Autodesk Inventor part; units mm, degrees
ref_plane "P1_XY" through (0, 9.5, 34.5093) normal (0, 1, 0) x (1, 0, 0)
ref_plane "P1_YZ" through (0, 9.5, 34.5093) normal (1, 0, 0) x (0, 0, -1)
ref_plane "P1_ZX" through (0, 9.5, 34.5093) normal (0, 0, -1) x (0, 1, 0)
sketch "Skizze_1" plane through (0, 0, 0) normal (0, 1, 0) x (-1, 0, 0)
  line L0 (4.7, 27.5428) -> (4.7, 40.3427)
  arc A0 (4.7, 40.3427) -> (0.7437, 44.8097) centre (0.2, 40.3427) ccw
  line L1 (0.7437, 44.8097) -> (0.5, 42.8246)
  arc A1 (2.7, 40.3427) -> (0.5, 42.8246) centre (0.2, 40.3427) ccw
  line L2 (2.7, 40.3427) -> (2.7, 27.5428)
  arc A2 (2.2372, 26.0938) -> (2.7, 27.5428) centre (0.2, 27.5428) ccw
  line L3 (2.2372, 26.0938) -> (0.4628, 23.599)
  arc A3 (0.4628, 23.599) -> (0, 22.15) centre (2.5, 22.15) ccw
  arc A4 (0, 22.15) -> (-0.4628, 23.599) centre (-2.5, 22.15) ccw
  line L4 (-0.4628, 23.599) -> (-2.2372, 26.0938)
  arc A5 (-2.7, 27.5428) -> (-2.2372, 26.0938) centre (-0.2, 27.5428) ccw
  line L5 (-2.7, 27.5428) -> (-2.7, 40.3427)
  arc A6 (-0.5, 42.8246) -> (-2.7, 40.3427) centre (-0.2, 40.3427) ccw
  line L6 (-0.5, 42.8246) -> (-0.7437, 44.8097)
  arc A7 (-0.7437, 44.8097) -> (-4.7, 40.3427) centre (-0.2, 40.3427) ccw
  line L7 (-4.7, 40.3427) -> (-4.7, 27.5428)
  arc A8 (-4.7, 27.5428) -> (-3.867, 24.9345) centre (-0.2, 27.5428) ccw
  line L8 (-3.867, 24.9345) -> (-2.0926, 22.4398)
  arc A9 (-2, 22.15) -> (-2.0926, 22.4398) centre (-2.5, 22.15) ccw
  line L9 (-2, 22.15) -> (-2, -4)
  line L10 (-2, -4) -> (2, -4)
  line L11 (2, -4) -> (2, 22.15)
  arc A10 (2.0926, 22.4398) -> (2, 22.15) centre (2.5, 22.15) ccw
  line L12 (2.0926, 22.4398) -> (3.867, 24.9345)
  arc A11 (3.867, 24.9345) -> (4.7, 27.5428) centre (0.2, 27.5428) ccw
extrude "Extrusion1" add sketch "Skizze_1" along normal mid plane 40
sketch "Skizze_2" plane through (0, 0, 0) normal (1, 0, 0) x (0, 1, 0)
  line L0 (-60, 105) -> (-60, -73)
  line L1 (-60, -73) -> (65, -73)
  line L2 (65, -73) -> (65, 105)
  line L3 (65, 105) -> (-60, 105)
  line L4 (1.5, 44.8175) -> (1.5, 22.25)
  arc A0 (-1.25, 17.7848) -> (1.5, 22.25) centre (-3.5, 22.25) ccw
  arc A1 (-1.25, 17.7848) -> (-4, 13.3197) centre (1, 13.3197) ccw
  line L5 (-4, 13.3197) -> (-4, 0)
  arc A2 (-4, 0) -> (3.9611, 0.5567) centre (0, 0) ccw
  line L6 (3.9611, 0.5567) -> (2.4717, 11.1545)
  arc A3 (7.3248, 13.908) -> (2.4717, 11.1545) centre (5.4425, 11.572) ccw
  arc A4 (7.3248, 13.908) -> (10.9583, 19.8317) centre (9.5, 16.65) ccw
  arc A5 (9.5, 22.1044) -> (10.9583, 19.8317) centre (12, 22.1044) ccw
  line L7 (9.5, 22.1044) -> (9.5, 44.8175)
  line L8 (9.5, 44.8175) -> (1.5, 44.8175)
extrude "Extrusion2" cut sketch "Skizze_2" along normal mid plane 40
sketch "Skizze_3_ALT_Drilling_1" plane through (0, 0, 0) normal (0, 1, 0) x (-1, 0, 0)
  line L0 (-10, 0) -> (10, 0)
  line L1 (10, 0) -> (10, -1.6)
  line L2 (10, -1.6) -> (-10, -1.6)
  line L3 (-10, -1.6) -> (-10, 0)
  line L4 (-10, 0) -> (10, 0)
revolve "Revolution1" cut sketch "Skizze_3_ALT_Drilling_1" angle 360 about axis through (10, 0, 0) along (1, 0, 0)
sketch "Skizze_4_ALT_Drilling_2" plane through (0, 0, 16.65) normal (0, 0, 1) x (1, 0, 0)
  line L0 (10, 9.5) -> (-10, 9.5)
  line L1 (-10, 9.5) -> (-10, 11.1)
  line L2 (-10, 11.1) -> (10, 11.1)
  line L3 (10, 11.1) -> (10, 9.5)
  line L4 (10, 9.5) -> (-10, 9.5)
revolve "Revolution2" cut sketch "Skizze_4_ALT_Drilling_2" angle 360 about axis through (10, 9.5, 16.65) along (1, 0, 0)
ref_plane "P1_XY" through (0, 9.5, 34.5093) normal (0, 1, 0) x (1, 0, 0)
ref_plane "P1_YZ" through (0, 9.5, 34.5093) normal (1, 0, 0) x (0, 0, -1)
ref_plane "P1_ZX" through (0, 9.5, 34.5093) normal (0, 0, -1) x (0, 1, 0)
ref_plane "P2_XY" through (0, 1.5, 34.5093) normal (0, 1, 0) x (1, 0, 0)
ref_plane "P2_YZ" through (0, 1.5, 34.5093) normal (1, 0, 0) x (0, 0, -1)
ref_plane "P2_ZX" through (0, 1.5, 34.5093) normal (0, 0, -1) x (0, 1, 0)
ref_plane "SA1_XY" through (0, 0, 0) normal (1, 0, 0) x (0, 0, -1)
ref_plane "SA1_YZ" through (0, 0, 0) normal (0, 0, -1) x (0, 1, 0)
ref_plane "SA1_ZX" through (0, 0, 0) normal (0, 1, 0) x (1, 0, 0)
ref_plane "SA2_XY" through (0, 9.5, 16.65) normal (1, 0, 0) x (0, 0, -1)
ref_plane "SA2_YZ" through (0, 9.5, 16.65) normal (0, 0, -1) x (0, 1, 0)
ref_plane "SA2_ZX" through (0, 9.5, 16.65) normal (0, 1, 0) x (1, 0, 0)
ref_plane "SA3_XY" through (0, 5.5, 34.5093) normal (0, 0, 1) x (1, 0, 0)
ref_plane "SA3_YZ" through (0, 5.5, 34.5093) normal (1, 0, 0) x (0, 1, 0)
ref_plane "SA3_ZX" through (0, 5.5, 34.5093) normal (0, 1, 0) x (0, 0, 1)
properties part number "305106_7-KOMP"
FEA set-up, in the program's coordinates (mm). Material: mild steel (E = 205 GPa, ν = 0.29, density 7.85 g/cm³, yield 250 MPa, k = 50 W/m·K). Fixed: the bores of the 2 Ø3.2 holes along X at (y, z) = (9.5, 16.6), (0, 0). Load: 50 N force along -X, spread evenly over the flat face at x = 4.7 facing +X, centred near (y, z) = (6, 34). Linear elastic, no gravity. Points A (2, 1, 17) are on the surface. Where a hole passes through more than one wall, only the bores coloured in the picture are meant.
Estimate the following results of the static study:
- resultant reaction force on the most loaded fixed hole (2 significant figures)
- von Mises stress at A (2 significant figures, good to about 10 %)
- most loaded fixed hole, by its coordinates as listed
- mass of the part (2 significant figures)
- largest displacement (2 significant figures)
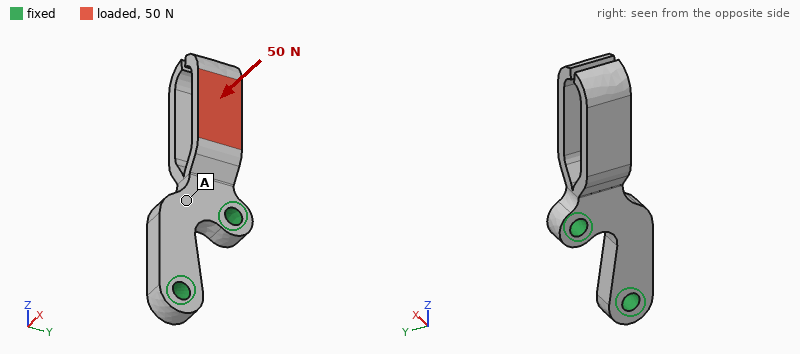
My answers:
64 N
13 MPa
(9.5, 16.6)
13 g
89 µm
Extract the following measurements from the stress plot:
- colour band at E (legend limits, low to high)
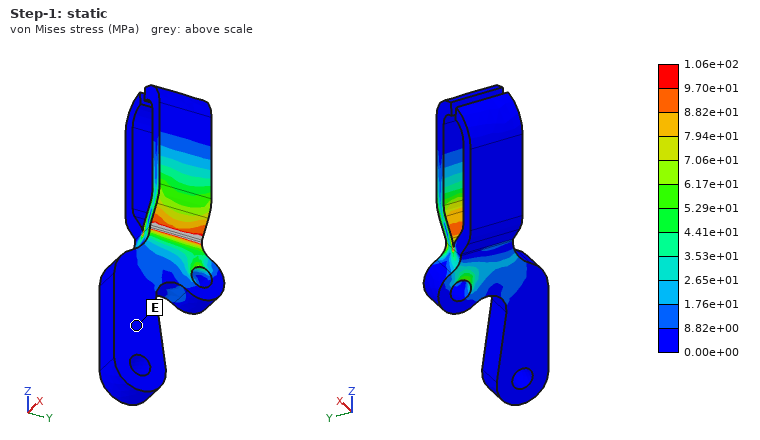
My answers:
0.00e+00 to 8.82e+00 MPa
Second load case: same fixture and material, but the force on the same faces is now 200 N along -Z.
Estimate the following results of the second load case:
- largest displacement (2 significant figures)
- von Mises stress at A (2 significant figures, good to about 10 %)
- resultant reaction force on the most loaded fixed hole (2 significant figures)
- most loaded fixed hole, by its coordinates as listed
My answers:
90 µm
21 MPa
140 N
(9.5, 16.6)
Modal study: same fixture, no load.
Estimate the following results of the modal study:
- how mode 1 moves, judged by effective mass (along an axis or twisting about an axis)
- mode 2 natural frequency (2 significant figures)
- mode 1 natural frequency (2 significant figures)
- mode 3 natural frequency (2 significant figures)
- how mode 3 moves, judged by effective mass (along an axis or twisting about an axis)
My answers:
along X
2700 Hz
2600 Hz
6600 Hz
along Y
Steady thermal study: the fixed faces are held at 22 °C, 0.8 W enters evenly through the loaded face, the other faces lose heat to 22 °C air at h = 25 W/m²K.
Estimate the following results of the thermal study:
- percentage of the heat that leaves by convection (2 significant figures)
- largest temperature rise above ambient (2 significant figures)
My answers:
16 %
14 K
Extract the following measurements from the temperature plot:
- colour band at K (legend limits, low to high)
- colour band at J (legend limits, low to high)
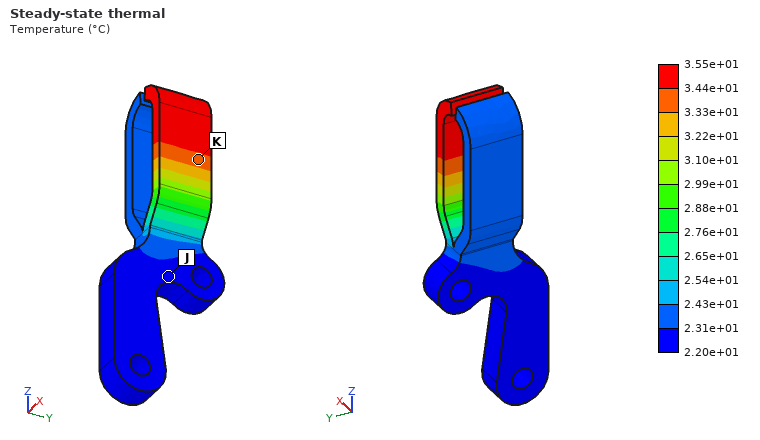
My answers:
3.33e+01 to 3.44e+01 °C
2.20e+01 to 2.31e+01 °C
